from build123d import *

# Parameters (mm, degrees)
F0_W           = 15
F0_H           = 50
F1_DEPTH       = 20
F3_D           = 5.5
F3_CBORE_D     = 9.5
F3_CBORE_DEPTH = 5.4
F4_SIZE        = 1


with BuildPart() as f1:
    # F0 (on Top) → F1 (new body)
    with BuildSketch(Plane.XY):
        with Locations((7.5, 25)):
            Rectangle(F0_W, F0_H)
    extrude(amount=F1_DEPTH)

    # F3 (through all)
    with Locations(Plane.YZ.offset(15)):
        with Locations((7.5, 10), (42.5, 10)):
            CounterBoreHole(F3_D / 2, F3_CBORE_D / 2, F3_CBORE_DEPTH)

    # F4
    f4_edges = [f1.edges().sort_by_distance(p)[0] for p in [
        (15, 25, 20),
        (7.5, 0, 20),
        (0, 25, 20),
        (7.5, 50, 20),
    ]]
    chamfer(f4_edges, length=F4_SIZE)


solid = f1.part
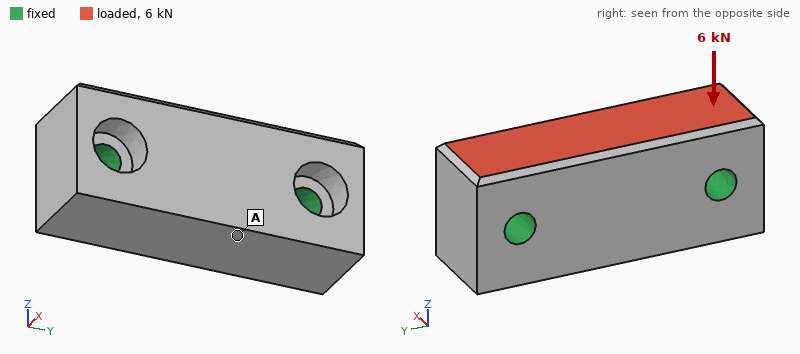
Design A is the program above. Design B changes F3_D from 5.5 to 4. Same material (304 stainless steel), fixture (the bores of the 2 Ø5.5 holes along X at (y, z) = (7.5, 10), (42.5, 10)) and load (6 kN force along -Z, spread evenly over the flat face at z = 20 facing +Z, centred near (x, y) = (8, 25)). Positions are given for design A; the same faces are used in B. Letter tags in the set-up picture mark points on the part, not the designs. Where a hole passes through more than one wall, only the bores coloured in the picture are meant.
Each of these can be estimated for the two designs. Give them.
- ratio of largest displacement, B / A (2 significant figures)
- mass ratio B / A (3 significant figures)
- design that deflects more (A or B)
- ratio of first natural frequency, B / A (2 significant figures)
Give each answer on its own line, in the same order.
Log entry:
1.3
1.02
B
0.87
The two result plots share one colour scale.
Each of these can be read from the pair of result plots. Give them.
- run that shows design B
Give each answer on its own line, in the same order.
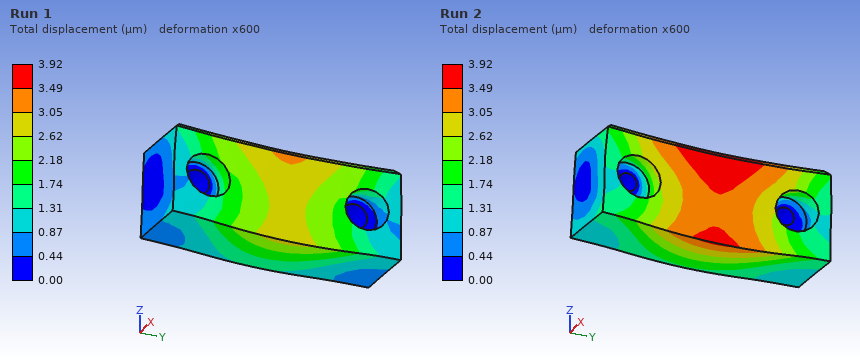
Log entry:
Run 2
